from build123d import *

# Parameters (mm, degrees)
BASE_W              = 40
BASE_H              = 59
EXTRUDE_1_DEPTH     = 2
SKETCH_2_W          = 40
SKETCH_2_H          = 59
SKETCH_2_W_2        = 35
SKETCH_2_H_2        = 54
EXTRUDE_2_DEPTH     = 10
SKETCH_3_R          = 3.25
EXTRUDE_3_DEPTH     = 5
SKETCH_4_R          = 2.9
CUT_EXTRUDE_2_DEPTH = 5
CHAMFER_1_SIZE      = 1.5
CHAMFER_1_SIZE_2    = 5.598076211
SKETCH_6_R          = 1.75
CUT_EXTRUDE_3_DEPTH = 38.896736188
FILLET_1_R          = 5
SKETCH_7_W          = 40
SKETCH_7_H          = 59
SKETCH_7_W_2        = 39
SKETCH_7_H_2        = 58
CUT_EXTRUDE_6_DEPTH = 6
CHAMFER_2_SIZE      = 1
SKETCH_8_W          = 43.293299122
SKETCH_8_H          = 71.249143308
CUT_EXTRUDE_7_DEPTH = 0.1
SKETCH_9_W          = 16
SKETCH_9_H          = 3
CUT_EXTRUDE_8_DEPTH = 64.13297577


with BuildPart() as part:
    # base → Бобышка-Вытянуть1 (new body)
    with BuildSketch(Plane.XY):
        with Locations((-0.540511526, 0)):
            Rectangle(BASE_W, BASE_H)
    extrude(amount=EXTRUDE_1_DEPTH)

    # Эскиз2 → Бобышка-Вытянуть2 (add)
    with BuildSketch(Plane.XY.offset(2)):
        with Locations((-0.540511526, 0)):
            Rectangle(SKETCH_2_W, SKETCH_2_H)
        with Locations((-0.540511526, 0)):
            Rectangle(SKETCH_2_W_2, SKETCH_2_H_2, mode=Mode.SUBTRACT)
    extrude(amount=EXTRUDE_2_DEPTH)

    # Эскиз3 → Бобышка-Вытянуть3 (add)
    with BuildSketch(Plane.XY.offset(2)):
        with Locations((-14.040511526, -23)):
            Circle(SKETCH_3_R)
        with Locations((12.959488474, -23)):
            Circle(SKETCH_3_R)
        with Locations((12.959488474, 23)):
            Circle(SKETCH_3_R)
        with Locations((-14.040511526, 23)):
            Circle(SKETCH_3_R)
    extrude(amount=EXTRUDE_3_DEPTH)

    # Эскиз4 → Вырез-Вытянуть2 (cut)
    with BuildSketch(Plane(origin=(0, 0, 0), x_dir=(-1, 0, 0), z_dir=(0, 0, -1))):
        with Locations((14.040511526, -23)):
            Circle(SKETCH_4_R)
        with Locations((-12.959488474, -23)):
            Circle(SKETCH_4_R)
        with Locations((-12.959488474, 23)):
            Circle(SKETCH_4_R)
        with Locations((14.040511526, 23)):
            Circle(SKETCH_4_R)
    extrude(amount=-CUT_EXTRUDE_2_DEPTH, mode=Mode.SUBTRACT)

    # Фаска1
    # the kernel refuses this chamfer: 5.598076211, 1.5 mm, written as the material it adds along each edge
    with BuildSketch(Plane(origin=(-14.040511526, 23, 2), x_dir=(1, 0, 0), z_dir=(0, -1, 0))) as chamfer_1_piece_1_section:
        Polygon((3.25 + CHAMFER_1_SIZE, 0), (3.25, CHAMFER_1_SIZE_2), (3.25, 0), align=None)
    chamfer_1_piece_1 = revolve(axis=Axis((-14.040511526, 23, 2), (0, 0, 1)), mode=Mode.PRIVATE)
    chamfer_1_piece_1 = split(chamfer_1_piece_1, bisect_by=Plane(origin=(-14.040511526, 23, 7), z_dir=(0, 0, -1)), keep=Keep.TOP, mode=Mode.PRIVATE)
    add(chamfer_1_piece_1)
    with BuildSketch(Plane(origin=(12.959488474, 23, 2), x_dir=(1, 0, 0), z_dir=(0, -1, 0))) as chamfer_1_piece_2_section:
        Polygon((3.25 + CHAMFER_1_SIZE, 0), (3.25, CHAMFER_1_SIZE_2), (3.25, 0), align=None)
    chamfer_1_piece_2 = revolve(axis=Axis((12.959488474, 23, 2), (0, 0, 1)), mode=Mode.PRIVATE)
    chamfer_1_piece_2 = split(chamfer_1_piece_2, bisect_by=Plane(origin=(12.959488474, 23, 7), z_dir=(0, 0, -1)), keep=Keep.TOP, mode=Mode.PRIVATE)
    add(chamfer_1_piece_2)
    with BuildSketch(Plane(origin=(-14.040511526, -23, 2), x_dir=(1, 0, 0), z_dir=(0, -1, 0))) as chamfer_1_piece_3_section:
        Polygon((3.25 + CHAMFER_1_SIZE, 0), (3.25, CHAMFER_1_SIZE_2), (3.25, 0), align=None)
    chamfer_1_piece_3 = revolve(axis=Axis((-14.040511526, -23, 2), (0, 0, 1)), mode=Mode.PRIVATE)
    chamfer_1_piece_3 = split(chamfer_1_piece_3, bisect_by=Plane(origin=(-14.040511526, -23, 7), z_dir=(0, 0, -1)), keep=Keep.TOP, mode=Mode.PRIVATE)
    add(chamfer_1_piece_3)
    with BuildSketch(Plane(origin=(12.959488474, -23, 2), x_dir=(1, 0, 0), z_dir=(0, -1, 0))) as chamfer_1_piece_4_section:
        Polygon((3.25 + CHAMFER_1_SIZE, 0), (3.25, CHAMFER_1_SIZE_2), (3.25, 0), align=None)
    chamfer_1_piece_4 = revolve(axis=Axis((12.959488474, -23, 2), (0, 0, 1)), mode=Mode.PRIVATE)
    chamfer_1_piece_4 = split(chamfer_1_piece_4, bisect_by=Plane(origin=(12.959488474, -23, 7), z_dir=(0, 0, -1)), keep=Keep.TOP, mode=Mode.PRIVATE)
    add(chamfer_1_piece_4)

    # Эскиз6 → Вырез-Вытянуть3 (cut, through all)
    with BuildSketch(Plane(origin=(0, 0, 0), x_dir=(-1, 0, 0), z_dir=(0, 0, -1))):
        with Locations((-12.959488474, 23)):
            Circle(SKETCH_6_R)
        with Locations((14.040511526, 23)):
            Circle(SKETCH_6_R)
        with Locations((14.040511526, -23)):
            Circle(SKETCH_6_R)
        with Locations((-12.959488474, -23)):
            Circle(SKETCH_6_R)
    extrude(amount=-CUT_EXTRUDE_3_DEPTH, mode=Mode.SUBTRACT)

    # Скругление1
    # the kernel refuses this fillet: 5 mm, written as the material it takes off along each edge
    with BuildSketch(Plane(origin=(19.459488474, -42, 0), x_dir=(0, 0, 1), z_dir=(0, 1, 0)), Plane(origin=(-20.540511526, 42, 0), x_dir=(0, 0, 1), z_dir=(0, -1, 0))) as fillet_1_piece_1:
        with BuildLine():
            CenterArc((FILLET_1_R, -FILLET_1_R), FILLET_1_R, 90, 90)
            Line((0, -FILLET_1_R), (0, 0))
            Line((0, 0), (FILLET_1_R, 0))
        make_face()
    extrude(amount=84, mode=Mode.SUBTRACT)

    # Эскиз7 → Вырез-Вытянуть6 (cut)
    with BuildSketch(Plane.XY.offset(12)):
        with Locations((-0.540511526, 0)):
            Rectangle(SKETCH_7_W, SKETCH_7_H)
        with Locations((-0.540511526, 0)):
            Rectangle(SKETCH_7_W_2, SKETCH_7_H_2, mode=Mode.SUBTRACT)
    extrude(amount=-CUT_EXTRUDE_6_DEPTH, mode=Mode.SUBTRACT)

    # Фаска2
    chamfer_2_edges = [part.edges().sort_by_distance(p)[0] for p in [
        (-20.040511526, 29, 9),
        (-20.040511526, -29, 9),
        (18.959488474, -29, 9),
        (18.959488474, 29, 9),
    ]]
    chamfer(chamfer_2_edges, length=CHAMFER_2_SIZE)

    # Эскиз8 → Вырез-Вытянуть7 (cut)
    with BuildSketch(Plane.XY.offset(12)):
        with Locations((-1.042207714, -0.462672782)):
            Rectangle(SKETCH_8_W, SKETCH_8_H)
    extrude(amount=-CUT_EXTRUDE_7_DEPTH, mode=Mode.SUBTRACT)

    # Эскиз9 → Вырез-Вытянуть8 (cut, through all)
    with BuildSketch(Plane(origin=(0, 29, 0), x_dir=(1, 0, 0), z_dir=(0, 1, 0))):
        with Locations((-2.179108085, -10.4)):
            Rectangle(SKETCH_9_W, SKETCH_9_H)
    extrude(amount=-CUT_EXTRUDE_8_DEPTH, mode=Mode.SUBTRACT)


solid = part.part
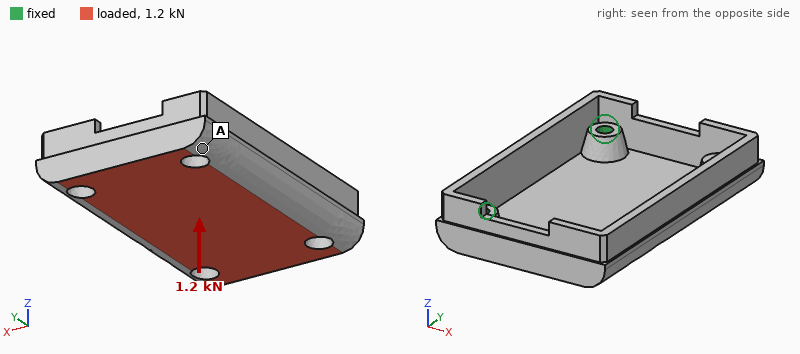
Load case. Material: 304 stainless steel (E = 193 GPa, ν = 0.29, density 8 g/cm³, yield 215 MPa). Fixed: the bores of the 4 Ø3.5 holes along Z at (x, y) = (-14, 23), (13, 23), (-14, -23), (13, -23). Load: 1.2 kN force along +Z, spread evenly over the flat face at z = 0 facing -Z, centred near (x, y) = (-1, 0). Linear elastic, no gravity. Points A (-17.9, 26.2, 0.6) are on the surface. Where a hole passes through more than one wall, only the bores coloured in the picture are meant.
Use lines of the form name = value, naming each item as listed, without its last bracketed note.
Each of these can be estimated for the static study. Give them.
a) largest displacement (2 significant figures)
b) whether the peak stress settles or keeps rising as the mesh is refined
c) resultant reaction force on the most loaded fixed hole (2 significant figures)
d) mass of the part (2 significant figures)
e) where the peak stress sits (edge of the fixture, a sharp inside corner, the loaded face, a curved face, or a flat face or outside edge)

largest displacement = 32 µm
whether the peak stress settles or keeps rising as the mesh is refined = keeps rising
resultant reaction force on the most loaded fixed hole = 350 N
mass of the part = 67 g
where the peak stress sits = edge of the fixture
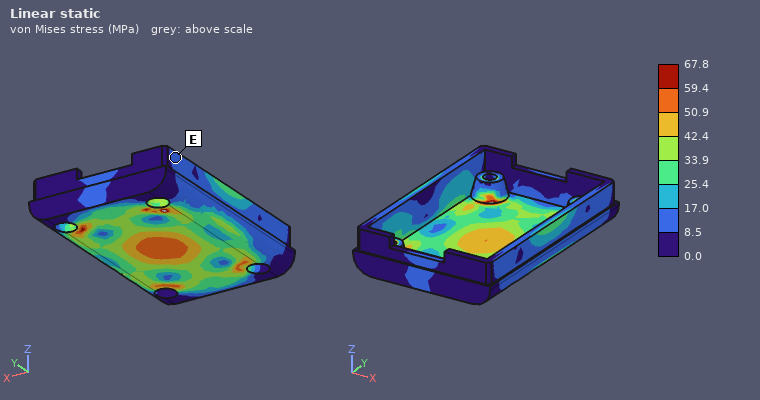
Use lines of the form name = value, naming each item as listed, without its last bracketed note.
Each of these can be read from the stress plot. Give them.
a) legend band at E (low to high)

legend band at E = 8.5 to 17.0 MPa
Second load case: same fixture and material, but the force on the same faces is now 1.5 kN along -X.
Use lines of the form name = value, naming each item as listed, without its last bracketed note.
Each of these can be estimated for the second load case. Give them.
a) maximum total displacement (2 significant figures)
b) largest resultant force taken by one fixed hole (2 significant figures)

maximum total displacement = 4.1 µm
largest resultant force taken by one fixed hole = 390 N
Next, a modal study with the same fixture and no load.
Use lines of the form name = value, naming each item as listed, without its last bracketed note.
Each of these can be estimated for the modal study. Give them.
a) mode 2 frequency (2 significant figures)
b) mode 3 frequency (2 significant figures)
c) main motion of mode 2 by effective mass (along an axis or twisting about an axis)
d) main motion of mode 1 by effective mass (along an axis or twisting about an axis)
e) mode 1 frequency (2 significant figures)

mode 2 frequency = 9000 Hz
mode 3 frequency = 9700 Hz
main motion of mode 2 by effective mass = along X
main motion of mode 1 by effective mass = along Z
mode 1 frequency = 6800 Hz
